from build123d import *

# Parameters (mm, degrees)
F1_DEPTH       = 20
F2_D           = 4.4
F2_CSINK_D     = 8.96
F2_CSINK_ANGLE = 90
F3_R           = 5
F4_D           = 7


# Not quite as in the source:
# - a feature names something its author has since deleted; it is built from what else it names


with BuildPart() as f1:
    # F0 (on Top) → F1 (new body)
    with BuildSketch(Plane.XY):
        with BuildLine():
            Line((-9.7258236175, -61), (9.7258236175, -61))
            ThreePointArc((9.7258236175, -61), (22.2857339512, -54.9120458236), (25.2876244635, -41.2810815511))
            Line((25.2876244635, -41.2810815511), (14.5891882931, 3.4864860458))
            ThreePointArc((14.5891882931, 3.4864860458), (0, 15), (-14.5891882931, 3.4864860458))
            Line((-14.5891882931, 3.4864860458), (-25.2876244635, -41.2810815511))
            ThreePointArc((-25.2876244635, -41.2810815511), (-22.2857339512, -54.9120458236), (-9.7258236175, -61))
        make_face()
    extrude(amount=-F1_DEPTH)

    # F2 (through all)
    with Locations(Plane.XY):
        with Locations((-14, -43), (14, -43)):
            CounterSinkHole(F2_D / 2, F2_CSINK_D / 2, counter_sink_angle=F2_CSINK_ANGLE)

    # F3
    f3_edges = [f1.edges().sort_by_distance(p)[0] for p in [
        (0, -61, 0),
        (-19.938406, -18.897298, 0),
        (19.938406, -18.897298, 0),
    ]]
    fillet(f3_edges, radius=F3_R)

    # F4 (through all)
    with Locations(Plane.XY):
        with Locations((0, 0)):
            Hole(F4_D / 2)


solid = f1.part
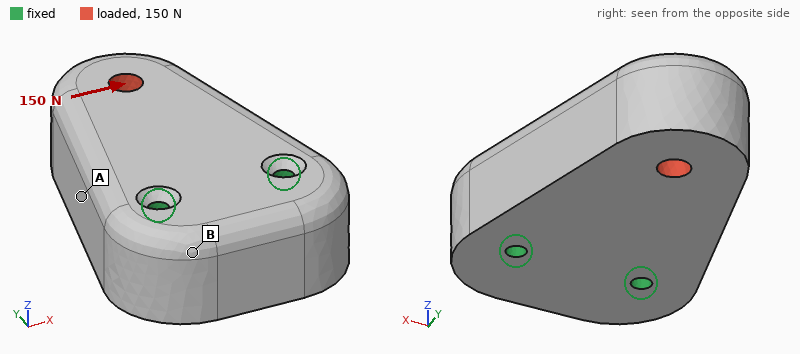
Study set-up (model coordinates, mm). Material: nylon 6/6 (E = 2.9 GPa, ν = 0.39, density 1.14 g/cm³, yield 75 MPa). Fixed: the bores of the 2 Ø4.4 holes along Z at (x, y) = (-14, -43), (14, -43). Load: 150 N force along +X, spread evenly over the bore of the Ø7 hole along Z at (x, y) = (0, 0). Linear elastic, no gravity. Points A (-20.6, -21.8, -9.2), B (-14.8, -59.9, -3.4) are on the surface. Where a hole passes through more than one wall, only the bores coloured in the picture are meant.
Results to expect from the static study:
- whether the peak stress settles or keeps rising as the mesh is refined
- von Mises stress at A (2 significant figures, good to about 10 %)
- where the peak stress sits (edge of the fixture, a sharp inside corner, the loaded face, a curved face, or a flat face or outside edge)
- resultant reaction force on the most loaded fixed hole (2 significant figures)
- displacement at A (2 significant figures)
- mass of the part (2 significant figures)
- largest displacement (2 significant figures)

keeps rising
0.64 MPa
edge of the fixture
230 N
10 µm
64 g
27 µm
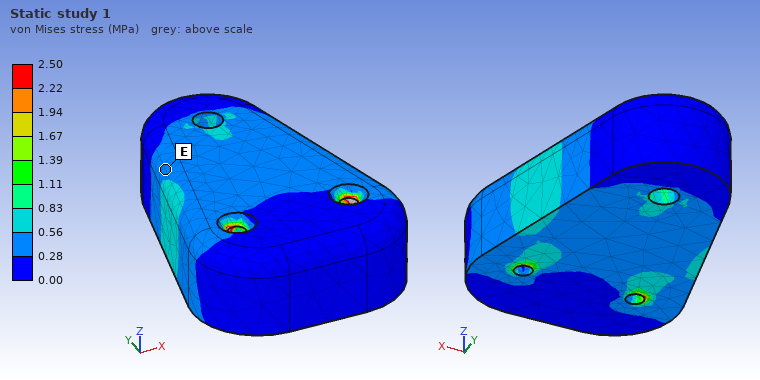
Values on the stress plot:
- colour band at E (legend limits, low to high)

0.28 to 0.56 MPa
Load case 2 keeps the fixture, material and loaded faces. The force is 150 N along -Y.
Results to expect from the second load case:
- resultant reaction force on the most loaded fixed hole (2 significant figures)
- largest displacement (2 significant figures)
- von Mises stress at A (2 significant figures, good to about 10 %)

76 N
4.8 µm
0.16 MPa
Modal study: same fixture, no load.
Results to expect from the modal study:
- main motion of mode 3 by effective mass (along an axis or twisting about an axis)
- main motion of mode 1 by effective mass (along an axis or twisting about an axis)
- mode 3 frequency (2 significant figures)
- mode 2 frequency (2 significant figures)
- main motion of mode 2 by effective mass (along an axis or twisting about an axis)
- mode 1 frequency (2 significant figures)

twisting about Y
along Z
4700 Hz
3000 Hz
along X
1600 Hz
